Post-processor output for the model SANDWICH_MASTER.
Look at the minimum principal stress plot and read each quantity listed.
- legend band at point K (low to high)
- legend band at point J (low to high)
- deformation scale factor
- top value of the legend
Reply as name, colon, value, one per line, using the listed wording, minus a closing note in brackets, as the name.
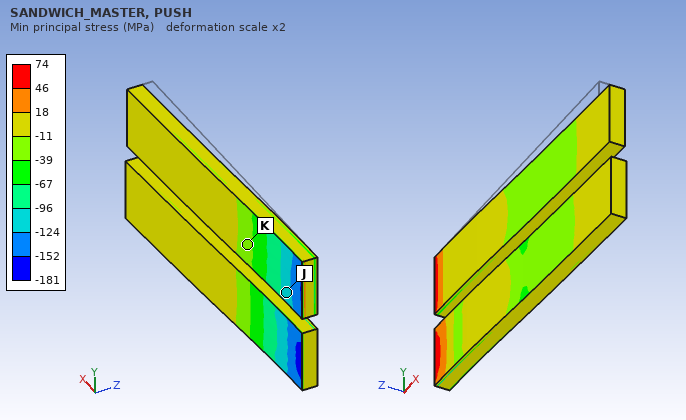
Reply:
legend band at point K: -39 to -11 MPa
legend band at point J: -124 to -96 MPa
deformation scale factor: 2
top value of the legend: 74 MPa
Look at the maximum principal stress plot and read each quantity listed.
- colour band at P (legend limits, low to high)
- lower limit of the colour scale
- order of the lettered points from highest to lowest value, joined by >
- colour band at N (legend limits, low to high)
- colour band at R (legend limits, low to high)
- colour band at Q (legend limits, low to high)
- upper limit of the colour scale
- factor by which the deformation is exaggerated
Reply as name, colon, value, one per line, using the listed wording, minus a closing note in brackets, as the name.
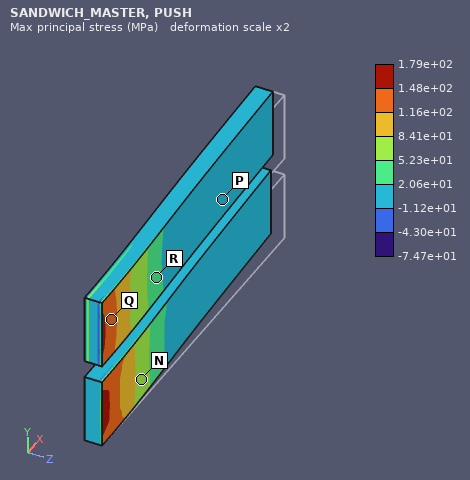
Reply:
colour band at P: -1.12e+01 to 2.06e+01 MPa
lower limit of the colour scale: -7.47e+01 MPa
order of the lettered points from highest to lowest value, joined by >: Q > N > R > P
colour band at N: 5.23e+01 to 8.41e+01 MPa
colour band at R: 2.06e+01 to 5.23e+01 MPa
colour band at Q: 1.16e+02 to 1.48e+02 MPa
upper limit of the colour scale: 1.79e+02 MPa
factor by which the deformation is exaggerated: 2
